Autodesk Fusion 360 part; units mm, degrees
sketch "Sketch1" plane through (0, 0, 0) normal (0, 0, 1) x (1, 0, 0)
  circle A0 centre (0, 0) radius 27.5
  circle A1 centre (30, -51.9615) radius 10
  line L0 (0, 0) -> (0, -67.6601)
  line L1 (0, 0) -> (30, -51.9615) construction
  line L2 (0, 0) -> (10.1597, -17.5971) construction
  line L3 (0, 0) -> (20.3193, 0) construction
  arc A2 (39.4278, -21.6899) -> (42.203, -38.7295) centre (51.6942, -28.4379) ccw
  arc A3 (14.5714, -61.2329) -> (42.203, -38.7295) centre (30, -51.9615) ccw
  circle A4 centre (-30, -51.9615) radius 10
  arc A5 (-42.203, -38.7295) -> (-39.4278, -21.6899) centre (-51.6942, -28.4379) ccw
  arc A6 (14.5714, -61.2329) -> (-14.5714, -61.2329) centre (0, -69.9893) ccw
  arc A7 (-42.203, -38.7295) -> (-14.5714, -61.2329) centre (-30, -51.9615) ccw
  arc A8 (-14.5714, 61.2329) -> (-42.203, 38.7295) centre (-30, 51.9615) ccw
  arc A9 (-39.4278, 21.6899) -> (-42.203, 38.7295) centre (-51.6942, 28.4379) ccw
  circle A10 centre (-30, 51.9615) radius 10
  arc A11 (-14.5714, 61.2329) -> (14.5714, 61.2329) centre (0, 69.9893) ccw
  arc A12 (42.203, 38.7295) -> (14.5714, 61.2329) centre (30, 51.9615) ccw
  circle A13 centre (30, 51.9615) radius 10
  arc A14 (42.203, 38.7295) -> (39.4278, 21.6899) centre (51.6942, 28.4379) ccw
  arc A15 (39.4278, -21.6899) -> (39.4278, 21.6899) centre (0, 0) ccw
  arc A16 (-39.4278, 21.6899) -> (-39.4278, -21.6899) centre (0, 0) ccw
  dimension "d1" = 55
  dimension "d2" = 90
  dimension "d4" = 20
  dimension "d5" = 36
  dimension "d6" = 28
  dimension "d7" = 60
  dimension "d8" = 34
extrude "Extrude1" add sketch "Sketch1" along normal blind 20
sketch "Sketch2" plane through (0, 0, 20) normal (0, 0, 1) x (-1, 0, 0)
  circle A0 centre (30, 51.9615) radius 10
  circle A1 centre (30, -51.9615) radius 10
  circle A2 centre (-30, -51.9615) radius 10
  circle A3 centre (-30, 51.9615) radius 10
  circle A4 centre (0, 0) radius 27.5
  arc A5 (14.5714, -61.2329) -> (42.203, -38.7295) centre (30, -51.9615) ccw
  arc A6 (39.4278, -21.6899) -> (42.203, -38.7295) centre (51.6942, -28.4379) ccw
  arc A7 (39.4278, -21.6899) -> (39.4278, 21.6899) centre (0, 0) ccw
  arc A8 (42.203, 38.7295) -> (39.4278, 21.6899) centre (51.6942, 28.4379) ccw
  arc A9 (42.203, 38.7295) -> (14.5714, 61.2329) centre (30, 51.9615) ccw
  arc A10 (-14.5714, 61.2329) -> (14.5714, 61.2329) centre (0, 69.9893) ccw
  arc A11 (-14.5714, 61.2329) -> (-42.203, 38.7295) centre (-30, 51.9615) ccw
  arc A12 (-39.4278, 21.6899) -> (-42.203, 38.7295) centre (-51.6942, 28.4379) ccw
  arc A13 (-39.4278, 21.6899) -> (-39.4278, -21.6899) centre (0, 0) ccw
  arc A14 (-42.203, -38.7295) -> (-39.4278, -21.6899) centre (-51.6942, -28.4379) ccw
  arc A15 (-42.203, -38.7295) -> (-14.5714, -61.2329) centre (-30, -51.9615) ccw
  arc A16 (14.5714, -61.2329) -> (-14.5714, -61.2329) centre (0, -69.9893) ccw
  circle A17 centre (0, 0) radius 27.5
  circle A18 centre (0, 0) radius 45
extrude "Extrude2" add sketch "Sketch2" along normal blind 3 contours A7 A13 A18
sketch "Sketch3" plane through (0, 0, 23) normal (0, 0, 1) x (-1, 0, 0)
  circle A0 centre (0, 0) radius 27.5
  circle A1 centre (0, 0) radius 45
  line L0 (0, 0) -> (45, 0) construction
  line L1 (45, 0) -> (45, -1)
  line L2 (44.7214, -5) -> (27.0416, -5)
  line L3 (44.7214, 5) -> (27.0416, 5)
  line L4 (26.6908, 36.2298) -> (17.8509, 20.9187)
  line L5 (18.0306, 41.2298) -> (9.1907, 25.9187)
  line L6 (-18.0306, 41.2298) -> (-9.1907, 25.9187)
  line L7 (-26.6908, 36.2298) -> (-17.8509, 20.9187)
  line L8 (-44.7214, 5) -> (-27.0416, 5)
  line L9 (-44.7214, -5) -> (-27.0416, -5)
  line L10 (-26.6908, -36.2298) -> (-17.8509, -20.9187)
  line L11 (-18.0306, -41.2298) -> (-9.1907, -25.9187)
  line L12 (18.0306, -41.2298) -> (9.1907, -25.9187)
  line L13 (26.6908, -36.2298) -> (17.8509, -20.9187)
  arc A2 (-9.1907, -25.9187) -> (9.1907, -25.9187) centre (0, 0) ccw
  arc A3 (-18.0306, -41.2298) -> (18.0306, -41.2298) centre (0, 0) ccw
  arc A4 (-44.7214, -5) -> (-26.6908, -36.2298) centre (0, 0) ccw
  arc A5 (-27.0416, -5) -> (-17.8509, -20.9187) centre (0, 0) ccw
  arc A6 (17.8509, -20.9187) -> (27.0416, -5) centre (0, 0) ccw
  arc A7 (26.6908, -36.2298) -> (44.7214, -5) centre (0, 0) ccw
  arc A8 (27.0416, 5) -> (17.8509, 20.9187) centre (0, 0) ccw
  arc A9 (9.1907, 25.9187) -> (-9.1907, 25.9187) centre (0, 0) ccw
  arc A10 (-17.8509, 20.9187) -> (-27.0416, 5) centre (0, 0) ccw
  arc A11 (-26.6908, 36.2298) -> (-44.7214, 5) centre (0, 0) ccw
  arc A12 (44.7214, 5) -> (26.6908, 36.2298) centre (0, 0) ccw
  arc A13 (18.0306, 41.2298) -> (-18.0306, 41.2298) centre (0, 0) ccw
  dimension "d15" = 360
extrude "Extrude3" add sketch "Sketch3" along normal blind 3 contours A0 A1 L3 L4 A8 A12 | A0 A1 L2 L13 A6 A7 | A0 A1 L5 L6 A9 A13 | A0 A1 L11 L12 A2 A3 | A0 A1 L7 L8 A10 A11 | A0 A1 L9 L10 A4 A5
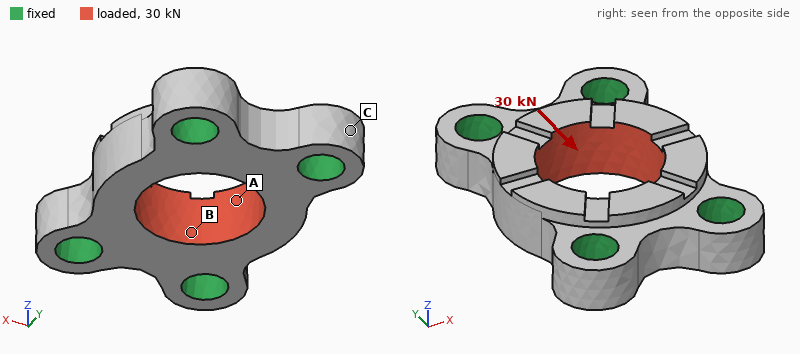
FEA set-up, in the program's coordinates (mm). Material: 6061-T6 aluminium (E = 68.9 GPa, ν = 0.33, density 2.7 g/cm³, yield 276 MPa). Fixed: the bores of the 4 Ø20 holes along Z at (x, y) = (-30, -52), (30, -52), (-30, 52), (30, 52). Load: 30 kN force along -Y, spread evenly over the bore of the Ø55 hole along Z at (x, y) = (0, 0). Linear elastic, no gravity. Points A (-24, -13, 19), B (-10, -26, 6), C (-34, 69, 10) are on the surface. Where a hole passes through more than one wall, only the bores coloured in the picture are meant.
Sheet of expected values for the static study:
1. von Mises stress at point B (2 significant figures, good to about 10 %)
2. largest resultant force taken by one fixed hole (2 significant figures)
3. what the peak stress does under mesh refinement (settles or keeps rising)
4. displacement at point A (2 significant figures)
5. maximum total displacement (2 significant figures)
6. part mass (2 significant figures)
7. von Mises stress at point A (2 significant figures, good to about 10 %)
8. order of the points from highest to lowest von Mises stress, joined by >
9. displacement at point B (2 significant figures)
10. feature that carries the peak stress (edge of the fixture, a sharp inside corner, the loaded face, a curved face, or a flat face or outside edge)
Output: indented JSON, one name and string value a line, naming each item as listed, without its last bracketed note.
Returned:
{
  "von Mises stress at point B": "6.9 MPa",
  "largest resultant force taken by one fixed hole": "7.9 kN",
  "what the peak stress does under mesh refinement": "keeps rising",
  "displacement at point A": "5.3 µm",
  "maximum total displacement": "6.7 µm",
  "part mass": "450 g",
  "von Mises stress at point A": "12 MPa",
  "order of the points from highest to lowest von Mises stress, joined by >": "A > B > C",
  "displacement at point B": "4.1 µm",
  "feature that carries the peak stress": "edge of the fixture"
}
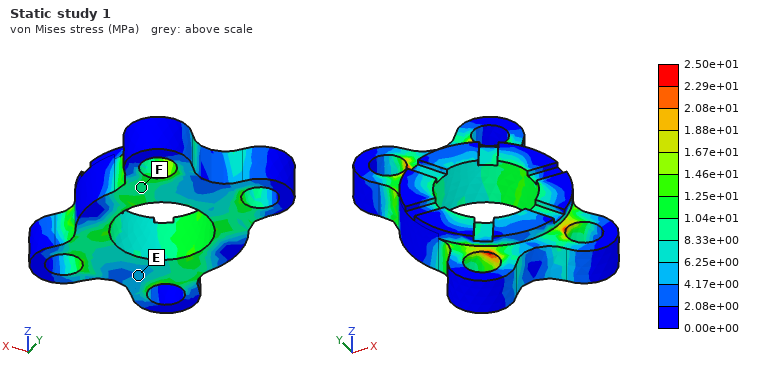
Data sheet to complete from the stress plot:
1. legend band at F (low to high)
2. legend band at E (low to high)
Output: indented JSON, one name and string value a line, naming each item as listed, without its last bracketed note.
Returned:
{
  "legend band at F": "8.33e+00 to 1.04e+01 MPa",
  "legend band at E": "4.17e+00 to 6.25e+00 MPa"
}
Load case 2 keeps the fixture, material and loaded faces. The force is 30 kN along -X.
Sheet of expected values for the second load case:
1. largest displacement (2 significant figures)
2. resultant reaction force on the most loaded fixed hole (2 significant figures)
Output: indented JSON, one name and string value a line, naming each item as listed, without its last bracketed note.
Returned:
{
  "largest displacement": "20 µm",
  "resultant reaction force on the most loaded fixed hole": "8.0 kN"
}
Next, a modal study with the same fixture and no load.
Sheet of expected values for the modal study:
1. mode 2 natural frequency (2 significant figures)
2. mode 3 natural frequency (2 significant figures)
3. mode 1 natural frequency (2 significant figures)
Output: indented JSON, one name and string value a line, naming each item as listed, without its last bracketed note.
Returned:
{
  "mode 2 natural frequency": "11 kHz",
  "mode 3 natural frequency": "15 kHz",
  "mode 1 natural frequency": "10 kHz"
}
